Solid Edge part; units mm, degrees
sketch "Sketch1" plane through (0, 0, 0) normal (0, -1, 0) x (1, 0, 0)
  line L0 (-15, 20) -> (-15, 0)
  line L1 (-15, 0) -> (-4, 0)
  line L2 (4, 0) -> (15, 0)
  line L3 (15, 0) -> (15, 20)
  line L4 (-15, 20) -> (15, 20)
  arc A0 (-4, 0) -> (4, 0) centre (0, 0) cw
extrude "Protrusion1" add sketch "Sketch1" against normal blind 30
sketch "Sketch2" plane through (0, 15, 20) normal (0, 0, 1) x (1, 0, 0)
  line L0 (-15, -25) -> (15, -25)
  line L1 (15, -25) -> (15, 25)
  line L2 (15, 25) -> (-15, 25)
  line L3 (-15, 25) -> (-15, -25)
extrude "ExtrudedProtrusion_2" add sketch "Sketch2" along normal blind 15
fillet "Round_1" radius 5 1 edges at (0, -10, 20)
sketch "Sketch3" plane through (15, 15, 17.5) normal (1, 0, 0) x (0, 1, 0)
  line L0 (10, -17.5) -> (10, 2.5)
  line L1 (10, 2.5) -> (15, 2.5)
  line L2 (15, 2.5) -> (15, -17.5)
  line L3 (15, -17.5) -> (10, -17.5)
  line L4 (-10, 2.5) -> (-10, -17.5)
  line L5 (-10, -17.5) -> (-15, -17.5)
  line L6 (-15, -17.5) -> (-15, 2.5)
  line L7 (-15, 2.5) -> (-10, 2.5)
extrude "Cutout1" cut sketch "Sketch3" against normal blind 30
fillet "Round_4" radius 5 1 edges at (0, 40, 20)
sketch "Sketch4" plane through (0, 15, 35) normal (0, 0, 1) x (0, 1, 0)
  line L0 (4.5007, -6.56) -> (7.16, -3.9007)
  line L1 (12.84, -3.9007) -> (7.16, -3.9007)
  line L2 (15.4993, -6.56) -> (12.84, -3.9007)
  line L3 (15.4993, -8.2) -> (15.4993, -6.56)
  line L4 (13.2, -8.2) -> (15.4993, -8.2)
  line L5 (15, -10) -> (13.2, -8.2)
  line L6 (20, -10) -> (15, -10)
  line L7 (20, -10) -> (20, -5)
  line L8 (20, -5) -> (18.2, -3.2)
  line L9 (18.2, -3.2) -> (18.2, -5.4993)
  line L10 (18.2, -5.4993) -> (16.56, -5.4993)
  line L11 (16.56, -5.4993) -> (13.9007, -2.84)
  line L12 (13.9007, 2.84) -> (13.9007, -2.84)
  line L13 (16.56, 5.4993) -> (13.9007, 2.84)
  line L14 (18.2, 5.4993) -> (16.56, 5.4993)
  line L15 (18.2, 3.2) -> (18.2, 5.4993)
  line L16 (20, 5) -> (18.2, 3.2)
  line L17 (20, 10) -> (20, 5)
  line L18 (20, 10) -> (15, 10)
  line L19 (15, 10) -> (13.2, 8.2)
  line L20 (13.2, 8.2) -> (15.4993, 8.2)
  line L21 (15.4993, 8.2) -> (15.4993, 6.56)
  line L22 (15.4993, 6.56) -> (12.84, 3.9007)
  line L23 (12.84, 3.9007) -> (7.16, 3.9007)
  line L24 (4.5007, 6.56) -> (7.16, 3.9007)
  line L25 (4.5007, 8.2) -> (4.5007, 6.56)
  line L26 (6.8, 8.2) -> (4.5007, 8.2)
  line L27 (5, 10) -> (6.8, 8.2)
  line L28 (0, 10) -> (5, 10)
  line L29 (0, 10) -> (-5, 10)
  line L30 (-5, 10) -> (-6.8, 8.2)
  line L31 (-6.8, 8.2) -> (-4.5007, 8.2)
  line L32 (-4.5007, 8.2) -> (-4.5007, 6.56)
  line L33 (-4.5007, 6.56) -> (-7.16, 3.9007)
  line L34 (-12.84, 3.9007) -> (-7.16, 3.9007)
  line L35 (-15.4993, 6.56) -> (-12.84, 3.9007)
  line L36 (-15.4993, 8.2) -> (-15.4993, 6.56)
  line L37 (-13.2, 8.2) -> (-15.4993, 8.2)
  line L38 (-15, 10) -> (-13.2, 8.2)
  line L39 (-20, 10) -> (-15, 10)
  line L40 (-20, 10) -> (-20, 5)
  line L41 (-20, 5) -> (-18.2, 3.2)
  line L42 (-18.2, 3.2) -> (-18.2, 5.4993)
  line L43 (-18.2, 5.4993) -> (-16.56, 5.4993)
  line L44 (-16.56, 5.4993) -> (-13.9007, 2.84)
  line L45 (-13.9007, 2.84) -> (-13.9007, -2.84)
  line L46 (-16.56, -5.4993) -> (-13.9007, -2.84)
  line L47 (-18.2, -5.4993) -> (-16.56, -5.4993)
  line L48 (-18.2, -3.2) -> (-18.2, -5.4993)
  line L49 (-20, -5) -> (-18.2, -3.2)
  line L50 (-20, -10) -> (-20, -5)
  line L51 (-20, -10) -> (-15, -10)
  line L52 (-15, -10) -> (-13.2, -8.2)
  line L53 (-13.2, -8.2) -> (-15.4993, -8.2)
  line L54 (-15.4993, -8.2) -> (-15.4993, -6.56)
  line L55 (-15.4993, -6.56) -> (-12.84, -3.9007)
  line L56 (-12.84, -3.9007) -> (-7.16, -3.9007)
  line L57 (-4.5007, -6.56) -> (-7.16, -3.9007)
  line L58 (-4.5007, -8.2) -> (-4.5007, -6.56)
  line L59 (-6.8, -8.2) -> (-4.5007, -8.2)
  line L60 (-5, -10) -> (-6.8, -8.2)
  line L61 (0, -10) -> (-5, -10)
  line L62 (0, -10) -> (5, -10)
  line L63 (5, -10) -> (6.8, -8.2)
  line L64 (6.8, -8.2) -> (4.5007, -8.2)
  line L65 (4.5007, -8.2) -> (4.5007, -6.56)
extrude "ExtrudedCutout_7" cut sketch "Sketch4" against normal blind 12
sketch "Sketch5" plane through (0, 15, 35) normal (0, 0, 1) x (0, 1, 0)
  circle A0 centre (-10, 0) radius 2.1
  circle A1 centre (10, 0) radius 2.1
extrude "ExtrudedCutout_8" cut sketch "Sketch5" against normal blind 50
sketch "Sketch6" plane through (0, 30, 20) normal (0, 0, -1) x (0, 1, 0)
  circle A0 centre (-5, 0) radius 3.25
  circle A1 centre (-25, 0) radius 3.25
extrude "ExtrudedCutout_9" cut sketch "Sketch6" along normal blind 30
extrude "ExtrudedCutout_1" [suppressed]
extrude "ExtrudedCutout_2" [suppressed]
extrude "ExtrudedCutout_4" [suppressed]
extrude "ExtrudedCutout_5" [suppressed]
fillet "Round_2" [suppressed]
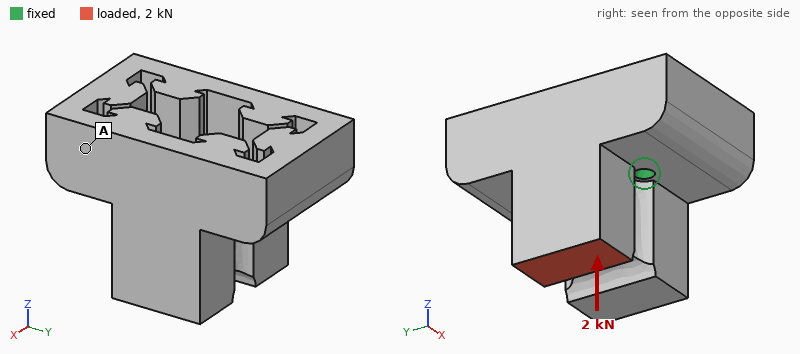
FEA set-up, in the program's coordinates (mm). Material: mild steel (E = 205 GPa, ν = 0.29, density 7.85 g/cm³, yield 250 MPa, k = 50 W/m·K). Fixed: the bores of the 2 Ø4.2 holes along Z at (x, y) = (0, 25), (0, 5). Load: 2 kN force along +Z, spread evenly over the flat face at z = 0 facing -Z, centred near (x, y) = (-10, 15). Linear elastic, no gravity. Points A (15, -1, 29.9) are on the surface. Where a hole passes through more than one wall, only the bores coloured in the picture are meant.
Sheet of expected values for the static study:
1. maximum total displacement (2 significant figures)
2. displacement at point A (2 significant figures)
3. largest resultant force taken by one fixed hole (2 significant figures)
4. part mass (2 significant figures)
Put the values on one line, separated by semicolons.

32 µm; 19 µm; 1.0 kN; 220 g
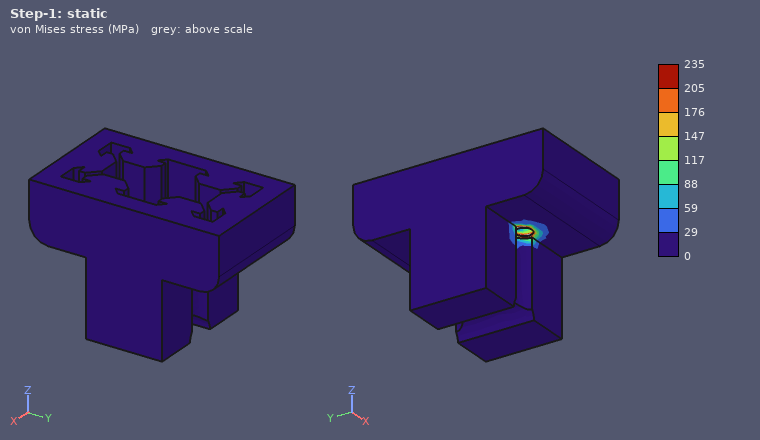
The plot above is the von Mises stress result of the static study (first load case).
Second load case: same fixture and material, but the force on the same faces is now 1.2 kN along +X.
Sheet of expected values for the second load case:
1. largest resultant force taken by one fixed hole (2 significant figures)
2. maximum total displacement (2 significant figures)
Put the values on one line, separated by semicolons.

600 N; 45 µm
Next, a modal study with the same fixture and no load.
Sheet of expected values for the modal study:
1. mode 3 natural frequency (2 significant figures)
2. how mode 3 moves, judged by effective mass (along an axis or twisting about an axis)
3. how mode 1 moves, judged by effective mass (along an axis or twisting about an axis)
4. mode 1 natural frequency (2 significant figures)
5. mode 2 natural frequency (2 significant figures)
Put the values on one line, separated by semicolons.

12 kHz; twisting about Z; twisting about Y; 3200 Hz; 8500 Hz
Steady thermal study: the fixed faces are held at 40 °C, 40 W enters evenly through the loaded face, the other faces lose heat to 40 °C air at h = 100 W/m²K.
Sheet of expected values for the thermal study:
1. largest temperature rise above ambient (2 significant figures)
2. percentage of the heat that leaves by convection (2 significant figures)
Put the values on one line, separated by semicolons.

69 K; 38 %
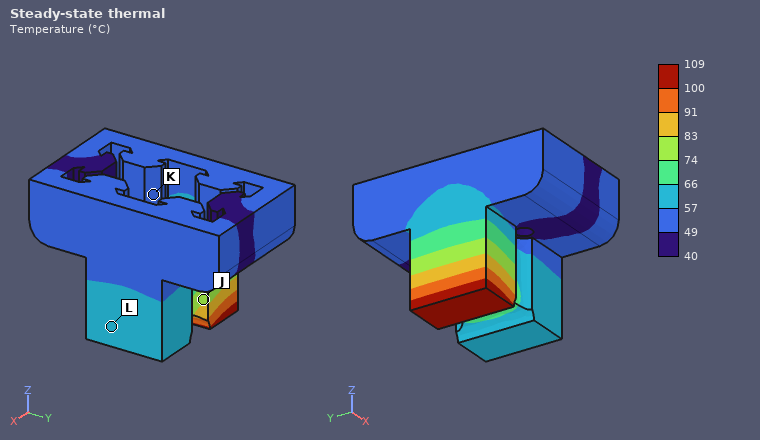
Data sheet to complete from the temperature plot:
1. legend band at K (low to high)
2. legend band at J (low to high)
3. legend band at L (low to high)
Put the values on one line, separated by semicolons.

49 to 57 °C; 74 to 83 °C; 57 to 66 °C
